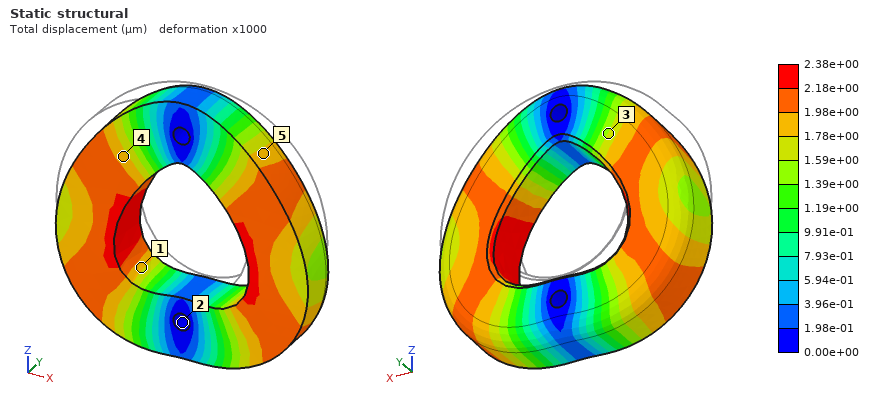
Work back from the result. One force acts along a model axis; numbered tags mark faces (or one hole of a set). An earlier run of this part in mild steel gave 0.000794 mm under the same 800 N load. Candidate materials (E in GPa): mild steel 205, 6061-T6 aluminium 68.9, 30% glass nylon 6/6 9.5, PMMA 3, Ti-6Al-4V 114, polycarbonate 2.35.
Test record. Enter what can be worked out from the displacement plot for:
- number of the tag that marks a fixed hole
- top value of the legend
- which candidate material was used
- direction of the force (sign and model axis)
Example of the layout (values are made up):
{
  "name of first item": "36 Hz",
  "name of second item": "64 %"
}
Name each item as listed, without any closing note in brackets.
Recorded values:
{
  "number of the tag that marks a fixed hole": "2",
  "top value of the legend": "2.38e+00 µm",
  "which candidate material was used": "6061-T6 aluminium",
  "direction of the force": "-Z"
}
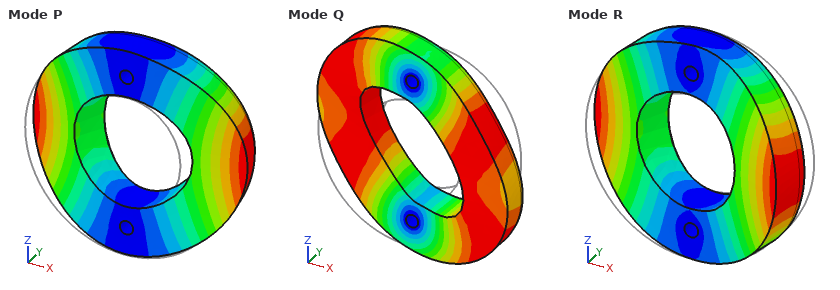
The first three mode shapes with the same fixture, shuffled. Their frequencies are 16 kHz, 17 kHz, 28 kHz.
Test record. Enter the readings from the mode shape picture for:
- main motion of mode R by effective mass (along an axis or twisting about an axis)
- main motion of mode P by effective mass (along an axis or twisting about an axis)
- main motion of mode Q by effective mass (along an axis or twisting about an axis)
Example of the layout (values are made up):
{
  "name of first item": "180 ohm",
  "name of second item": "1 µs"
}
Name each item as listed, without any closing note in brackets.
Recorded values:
{
  "main motion of mode R by effective mass": "twisting about Z",
  "main motion of mode P by effective mass": "along Y",
  "main motion of mode Q by effective mass": "twisting about Y"
}
